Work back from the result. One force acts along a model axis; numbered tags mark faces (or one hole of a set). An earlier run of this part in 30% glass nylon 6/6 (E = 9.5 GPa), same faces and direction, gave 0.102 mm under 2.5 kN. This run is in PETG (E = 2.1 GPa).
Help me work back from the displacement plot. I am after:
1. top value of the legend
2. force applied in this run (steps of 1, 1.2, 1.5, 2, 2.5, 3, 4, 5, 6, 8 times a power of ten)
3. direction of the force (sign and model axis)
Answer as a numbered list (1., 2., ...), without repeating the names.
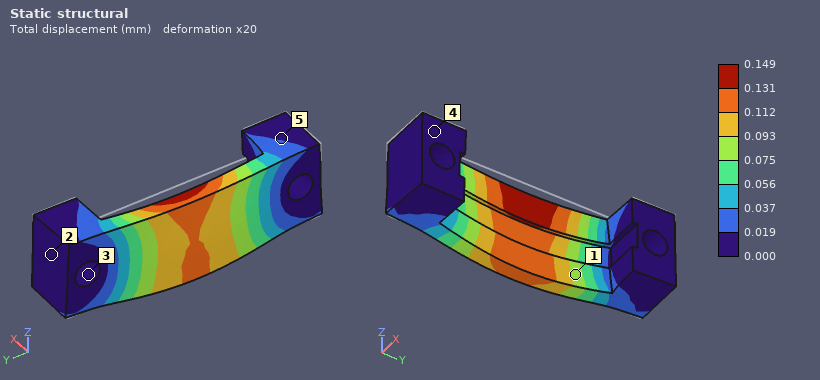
1. 0.149 mm
2. 800 N
3. -Z
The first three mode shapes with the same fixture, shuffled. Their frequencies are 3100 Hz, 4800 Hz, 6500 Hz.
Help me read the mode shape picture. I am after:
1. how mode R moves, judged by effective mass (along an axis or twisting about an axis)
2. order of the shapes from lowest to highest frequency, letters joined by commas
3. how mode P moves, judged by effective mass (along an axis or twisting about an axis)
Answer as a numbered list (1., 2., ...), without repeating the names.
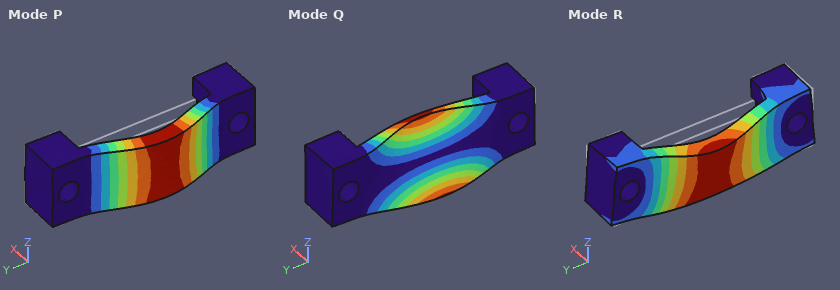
1. along Z
2. P, Q, R
3. along X
